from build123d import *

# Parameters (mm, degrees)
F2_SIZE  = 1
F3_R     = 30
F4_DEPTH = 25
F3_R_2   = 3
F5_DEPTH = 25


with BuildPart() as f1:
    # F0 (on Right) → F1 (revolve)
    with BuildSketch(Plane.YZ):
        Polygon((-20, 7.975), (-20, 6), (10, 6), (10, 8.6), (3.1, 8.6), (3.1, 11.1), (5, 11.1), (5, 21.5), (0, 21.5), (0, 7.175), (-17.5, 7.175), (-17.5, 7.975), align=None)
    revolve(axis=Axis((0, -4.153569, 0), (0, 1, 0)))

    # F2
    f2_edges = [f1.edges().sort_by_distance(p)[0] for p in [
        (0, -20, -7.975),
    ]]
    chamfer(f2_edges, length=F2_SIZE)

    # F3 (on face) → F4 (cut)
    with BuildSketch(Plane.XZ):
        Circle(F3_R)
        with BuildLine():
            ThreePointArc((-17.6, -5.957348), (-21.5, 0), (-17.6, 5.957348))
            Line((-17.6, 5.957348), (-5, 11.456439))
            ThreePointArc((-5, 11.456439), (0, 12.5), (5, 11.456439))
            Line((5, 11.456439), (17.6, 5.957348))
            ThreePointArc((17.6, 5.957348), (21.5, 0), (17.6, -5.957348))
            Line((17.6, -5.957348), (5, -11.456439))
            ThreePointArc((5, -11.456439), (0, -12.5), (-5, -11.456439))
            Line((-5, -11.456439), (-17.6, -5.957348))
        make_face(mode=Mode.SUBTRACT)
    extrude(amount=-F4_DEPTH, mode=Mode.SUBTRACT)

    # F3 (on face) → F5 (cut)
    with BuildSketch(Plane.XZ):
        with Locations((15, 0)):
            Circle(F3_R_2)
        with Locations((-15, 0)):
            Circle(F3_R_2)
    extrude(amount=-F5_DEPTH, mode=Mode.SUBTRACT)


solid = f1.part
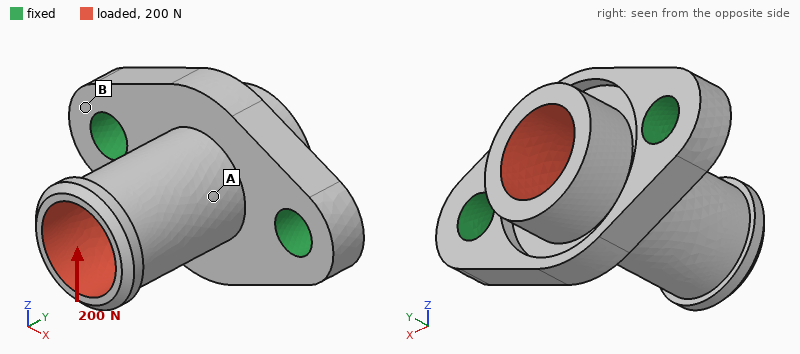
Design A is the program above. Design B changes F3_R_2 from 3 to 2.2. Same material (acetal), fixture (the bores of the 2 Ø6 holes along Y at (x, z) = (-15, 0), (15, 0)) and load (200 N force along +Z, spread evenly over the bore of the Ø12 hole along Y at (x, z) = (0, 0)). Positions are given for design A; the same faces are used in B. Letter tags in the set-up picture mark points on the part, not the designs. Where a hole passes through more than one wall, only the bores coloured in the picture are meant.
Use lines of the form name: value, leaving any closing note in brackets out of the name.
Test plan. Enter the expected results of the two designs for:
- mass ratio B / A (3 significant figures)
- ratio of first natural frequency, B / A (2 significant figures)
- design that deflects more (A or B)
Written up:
mass ratio B / A: 1.03
ratio of first natural frequency, B / A: 0.93
design that deflects more: B
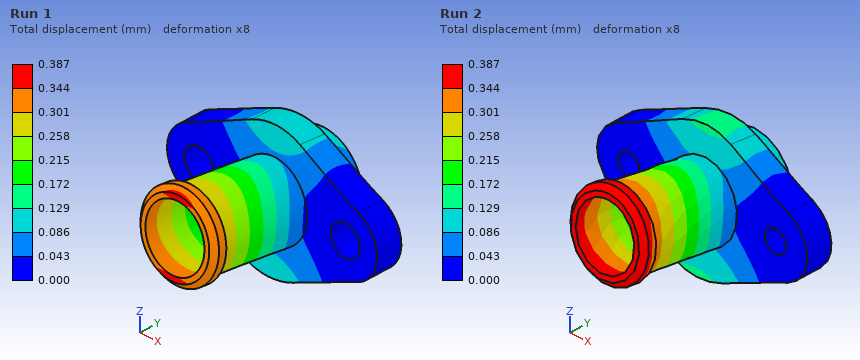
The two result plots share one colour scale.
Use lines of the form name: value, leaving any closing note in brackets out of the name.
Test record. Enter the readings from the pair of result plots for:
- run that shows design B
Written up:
run that shows design B: Run 2
